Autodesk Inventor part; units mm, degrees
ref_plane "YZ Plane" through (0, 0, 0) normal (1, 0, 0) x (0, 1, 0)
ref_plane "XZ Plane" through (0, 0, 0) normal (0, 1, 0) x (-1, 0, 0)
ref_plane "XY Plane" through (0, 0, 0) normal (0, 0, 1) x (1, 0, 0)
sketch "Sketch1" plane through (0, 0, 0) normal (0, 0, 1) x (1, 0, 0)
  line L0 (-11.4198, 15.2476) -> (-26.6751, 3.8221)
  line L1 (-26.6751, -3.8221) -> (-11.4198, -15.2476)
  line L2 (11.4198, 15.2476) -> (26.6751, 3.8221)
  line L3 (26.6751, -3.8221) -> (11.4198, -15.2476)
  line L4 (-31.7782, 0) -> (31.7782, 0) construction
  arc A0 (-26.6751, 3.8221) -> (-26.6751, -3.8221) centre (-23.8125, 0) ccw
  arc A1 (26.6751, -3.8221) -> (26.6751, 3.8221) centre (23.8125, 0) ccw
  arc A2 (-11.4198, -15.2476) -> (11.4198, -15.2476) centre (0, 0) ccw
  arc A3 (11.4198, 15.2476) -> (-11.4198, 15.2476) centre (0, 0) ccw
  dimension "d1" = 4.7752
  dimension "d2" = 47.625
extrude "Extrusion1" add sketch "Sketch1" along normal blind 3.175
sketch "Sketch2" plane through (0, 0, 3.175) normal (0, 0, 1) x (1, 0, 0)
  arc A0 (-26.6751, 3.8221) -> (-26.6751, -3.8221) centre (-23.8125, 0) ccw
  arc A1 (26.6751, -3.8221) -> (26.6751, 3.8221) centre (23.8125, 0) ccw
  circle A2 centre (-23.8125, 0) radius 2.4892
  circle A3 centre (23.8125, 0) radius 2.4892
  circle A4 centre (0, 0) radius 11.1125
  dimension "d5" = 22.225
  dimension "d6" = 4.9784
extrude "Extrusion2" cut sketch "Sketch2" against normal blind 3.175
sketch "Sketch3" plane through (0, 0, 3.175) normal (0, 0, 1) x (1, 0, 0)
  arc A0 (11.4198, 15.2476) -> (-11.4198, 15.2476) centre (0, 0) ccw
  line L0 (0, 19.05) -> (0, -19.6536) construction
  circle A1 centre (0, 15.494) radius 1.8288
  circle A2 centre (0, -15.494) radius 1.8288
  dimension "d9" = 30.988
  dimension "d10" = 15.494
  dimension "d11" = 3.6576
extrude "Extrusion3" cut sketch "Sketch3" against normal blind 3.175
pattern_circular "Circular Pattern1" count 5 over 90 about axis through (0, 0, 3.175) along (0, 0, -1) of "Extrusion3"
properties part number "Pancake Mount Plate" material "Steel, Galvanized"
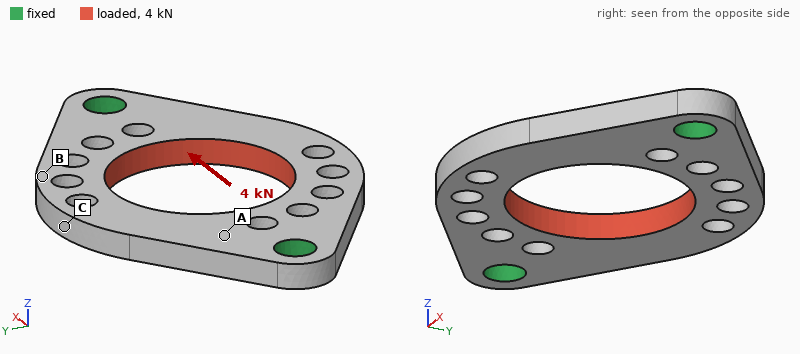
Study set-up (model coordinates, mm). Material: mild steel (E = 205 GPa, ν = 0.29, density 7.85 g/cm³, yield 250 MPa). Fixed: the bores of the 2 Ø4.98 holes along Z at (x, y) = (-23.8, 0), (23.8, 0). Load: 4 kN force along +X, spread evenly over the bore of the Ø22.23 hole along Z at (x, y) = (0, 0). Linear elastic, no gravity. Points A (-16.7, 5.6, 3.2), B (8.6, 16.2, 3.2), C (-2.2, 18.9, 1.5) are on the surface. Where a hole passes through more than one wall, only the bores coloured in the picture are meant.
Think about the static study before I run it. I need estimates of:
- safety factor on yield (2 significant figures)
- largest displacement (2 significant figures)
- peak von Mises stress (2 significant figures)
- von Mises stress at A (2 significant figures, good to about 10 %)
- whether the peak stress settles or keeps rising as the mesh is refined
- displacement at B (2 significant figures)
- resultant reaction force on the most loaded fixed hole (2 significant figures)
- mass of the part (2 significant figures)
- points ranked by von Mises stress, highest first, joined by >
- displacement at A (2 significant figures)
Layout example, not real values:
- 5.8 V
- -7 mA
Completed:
- 1.4
- 7.3 µm
- 170 MPa
- 39 MPa
- settles
- 5.5 µm
- 2.0 kN
- 22 g
- A > C > B
- 2.8 µm
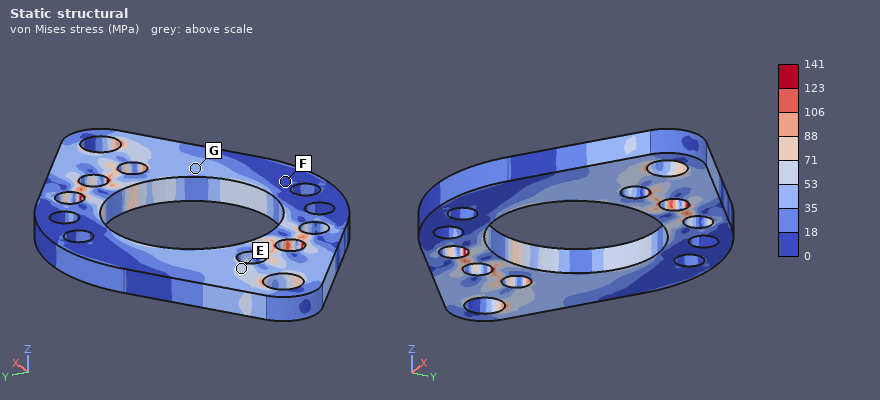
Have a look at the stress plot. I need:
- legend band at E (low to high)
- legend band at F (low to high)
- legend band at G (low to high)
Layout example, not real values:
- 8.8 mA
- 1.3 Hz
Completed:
- 53 to 71 MPa
- 0 to 18 MPa
- 35 to 53 MPa
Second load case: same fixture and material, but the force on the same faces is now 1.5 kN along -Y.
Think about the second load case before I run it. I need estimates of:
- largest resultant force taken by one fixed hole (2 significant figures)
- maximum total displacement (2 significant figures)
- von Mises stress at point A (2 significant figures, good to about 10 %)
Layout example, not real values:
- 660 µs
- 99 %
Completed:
- 750 N
- 4.8 µm
- 25 MPa
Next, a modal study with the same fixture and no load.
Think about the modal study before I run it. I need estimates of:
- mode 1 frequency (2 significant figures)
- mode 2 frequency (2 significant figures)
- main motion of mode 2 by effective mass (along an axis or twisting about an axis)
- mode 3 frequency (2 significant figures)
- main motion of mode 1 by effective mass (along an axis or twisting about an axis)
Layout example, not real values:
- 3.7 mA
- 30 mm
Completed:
- 5000 Hz
- 5500 Hz
- along Z
- 14 kHz
- twisting about X
